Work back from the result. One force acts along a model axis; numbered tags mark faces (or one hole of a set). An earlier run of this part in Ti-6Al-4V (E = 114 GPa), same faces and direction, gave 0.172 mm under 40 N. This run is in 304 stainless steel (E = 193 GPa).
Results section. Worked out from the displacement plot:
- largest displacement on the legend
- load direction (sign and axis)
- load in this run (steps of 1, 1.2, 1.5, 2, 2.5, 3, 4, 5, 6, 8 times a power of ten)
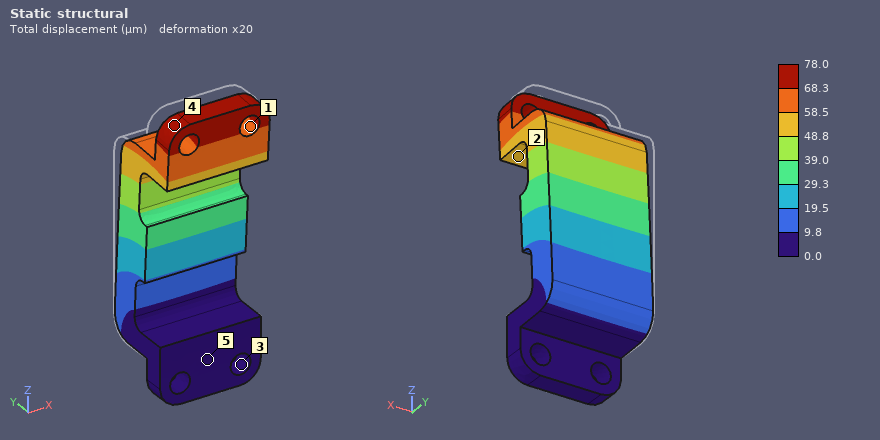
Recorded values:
78.0 µm
-Y
30 N
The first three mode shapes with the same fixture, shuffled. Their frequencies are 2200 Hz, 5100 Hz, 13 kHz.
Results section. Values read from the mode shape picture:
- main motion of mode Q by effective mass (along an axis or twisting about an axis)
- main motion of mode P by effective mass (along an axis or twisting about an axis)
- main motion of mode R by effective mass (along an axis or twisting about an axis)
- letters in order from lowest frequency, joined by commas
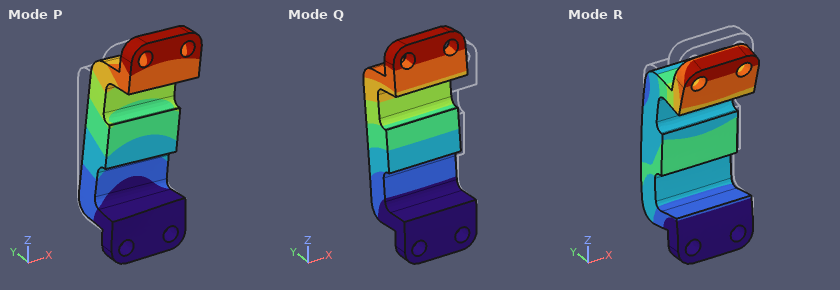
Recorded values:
along Y
along X
along Z
Q, P, R
